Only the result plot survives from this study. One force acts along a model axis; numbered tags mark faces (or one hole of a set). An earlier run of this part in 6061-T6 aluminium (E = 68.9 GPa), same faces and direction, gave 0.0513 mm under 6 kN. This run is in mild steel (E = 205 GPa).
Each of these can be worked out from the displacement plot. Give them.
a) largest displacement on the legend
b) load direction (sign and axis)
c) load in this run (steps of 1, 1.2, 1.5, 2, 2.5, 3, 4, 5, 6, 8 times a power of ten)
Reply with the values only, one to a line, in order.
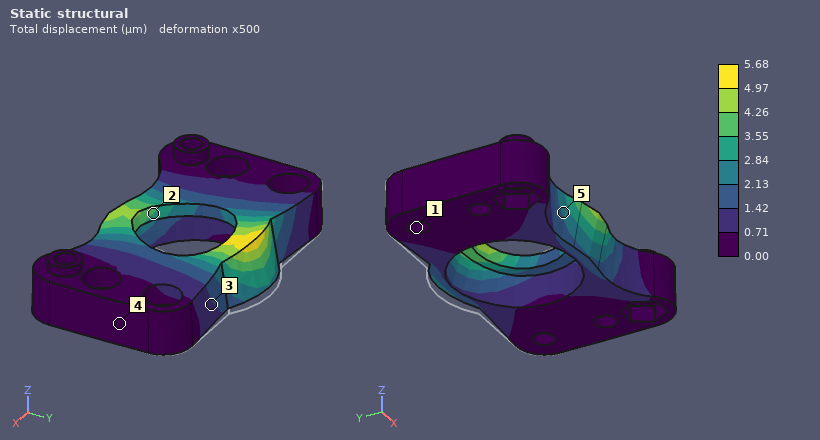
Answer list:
5.68 µm
-Y
2 kN
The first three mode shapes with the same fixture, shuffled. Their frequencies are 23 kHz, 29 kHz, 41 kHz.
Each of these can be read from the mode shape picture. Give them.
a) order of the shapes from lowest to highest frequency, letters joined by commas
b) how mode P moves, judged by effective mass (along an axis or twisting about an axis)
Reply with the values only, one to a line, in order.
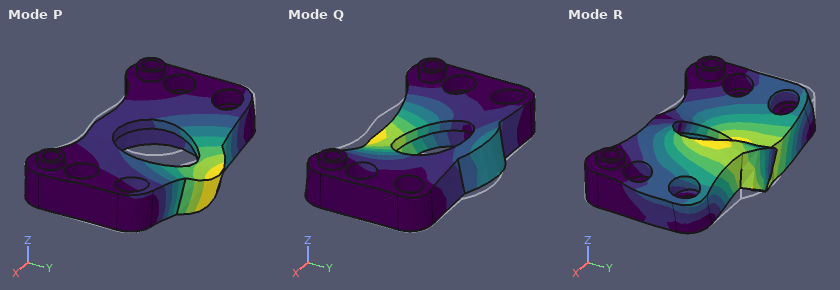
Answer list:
P, Q, R
along Z
